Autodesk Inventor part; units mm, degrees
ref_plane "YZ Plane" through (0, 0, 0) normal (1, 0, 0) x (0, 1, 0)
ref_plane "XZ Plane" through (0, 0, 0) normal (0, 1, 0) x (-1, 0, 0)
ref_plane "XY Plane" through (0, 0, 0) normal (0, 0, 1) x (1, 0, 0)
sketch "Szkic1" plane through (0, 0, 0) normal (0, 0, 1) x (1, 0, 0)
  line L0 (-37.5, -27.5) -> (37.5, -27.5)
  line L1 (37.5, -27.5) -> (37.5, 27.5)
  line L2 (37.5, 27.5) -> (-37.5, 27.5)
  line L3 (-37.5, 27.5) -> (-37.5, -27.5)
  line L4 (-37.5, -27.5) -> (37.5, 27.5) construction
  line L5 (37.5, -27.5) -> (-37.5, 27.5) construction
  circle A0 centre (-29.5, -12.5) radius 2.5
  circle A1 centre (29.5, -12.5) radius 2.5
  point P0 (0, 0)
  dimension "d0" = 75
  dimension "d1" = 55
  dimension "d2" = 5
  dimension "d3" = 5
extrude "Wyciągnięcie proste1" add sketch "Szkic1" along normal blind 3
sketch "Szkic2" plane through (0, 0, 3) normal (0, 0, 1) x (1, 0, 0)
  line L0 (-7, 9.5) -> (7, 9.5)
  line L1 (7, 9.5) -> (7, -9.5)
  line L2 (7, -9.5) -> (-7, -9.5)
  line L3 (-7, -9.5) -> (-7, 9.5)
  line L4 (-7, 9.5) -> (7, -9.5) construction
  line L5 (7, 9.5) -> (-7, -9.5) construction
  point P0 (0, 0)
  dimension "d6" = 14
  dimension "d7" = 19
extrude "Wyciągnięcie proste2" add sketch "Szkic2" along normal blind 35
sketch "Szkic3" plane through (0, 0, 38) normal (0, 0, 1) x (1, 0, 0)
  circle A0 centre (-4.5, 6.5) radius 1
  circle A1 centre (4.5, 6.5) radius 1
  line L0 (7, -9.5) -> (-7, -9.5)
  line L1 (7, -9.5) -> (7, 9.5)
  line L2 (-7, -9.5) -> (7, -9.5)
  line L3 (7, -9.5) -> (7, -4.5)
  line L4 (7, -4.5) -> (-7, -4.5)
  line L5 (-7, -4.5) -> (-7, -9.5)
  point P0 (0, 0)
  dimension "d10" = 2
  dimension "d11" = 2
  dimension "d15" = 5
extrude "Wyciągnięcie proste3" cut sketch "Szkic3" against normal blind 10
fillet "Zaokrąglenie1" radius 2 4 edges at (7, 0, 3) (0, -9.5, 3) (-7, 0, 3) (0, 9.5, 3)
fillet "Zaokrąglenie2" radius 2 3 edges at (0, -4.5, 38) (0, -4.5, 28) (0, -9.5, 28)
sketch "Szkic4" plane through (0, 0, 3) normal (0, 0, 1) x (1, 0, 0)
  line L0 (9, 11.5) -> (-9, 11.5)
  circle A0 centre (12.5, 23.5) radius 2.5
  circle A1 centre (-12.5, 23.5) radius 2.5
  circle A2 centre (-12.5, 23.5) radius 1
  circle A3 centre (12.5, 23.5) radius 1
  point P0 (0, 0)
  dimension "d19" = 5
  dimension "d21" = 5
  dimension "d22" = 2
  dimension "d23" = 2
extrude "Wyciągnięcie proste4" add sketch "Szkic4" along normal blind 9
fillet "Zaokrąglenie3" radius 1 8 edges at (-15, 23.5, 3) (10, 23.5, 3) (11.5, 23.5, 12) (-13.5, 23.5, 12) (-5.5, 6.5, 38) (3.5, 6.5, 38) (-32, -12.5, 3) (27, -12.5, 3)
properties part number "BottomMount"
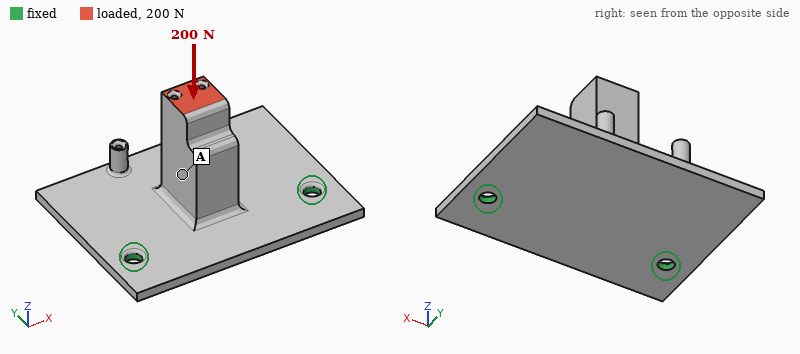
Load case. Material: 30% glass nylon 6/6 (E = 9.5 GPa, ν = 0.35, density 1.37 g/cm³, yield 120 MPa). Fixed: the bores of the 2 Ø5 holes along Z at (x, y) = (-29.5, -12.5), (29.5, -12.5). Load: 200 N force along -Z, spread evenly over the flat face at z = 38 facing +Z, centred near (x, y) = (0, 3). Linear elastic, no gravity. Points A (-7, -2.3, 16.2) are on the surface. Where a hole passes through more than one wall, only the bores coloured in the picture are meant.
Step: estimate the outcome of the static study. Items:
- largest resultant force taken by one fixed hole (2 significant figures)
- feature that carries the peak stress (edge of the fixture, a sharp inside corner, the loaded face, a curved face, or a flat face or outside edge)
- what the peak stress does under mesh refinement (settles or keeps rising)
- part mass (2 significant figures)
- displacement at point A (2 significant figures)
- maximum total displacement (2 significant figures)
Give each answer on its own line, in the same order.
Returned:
120 N
edge of the fixture
keeps rising
29 g
0.53 mm
1.1 mm
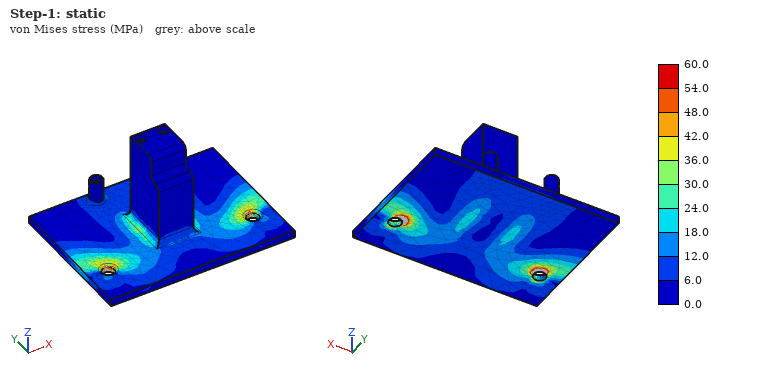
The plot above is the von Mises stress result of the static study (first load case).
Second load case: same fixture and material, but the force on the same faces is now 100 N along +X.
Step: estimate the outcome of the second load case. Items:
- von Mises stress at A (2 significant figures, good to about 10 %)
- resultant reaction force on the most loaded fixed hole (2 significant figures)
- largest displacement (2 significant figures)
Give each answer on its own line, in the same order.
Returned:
3.7 MPa
97 N
0.37 mm
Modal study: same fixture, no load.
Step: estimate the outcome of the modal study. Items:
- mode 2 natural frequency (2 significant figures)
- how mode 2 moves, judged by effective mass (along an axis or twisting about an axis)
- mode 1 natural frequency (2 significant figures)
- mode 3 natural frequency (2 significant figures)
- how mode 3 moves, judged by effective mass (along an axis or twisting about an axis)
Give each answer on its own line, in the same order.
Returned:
1200 Hz
along X
460 Hz
1300 Hz
along Z
